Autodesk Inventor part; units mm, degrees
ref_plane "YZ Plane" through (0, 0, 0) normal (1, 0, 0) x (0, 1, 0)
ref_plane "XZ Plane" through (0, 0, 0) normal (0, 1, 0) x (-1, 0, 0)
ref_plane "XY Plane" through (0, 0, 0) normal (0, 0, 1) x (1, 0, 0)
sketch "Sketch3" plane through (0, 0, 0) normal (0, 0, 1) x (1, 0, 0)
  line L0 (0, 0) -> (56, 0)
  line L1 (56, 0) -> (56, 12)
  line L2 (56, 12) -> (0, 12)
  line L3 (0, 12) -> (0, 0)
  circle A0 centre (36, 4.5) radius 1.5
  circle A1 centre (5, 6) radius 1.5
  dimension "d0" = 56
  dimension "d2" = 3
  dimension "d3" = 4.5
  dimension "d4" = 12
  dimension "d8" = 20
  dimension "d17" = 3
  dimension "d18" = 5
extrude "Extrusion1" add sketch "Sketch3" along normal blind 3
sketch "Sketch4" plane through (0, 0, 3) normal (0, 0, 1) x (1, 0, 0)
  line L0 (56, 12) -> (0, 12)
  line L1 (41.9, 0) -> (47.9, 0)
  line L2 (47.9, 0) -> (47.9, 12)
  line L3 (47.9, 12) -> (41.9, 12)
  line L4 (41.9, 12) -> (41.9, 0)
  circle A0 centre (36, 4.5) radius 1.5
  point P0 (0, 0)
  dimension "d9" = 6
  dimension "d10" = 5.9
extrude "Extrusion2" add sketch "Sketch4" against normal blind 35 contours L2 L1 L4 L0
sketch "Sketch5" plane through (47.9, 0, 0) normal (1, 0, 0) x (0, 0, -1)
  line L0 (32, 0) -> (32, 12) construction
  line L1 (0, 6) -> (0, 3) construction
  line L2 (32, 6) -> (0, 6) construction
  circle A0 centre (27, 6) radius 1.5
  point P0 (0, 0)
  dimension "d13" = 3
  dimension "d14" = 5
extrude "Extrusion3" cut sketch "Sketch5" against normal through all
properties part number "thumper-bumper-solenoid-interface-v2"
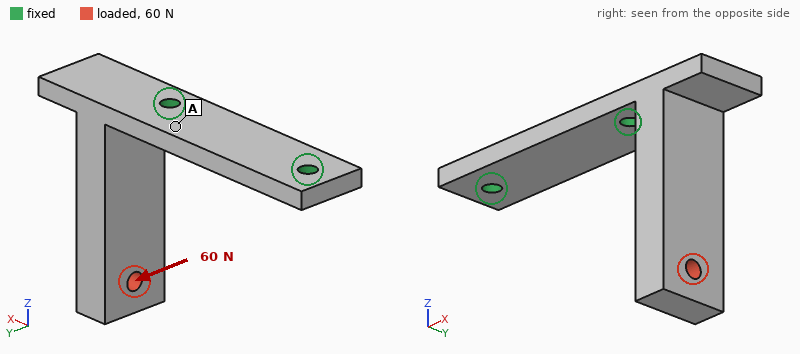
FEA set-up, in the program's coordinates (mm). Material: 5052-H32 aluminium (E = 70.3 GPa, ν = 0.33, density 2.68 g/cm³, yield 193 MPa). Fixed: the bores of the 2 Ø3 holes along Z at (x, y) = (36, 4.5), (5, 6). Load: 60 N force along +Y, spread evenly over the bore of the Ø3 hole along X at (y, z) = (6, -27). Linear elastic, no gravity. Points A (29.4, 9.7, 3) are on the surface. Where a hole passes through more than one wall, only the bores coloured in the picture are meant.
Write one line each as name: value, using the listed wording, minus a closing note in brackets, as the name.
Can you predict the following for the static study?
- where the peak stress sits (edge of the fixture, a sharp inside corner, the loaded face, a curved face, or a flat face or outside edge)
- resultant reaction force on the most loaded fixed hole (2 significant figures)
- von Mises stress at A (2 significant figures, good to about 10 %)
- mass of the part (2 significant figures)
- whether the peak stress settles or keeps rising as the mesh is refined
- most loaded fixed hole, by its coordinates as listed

where the peak stress sits: edge of the fixture
resultant reaction force on the most loaded fixed hole: 71 N
von Mises stress at A: 14 MPa
mass of the part: 11 g
whether the peak stress settles or keeps rising as the mesh is refined: keeps rising
most loaded fixed hole, by its coordinates as listed: (36, 4.5)
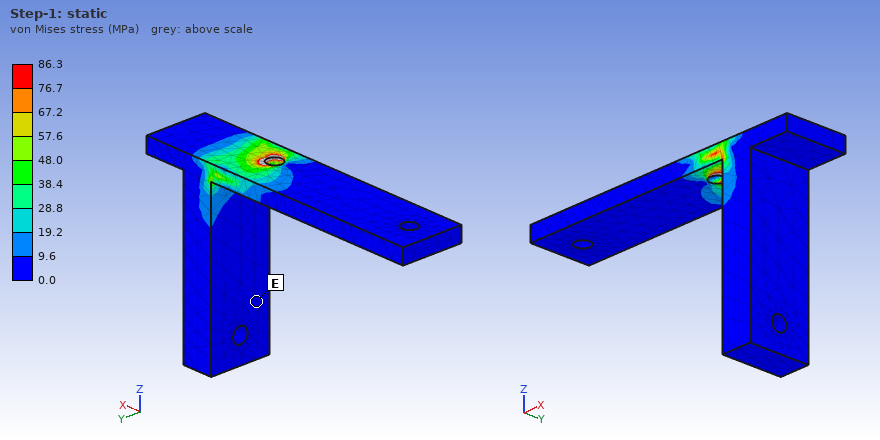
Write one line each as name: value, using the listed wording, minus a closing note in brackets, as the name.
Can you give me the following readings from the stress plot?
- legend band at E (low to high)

legend band at E: 0.0 to 9.6 MPa
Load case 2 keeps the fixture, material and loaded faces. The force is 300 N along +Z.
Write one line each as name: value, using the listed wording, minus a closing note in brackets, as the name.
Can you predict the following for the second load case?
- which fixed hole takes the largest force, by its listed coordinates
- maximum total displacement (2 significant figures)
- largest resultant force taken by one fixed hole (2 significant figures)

which fixed hole takes the largest force, by its listed coordinates: (36, 4.5)
maximum total displacement: 0.20 mm
largest resultant force taken by one fixed hole: 310 N
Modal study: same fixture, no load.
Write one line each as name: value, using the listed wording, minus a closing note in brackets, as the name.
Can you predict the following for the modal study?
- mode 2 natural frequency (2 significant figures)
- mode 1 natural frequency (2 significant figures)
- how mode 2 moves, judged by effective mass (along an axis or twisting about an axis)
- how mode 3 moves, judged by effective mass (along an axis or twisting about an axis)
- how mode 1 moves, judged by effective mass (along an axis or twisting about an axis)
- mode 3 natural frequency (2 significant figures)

mode 2 natural frequency: 2200 Hz
mode 1 natural frequency: 1500 Hz
how mode 2 moves, judged by effective mass: along Y
how mode 3 moves, judged by effective mass: along Z
how mode 1 moves, judged by effective mass: along X
mode 3 natural frequency: 9300 Hz
